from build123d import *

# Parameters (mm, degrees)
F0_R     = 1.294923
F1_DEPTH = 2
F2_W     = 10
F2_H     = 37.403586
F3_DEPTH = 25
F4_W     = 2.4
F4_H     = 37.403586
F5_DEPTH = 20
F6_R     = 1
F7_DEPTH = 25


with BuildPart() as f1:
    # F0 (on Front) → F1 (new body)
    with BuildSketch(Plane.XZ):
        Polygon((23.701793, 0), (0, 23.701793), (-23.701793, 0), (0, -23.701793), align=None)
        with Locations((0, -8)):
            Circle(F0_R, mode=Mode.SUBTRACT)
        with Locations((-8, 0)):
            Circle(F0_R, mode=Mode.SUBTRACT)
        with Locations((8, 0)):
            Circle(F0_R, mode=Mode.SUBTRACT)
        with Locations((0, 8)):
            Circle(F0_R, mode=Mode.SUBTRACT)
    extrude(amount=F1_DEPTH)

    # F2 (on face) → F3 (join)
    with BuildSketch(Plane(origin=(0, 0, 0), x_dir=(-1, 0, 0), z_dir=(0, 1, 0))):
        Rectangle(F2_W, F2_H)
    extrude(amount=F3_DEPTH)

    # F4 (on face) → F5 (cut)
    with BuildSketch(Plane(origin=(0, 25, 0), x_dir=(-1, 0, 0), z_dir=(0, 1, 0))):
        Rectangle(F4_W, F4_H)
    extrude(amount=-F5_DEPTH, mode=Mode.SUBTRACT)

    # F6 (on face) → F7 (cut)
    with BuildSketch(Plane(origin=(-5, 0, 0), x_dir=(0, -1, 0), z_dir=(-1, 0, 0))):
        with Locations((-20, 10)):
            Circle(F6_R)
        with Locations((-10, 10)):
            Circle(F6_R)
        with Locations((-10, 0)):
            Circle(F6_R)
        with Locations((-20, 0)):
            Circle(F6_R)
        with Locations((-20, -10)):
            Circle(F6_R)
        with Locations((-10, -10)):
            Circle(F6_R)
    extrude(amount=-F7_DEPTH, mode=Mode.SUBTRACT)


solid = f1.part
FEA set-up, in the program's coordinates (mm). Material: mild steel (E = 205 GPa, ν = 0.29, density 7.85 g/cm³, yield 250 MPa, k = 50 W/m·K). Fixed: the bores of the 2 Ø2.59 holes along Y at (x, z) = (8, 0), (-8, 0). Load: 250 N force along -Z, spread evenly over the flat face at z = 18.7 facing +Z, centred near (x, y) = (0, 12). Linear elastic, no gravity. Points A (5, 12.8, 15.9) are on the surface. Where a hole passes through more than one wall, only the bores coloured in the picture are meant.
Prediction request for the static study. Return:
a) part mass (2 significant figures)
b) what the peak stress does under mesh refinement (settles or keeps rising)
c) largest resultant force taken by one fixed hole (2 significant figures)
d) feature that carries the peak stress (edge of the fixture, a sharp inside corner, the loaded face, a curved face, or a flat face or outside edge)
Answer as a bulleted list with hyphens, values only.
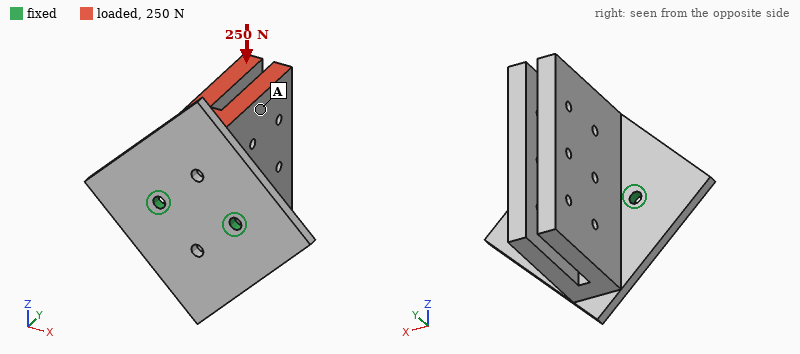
- 75 g
- keeps rising
- 130 N
- edge of the fixture
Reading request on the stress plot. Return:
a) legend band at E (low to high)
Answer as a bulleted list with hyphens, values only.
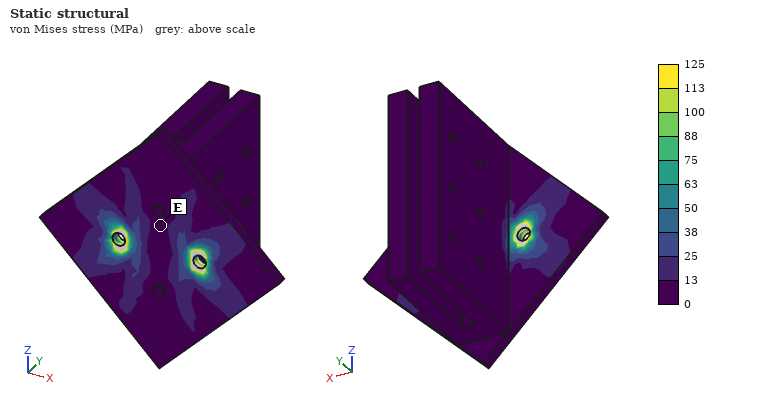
- 0 to 13 MPa
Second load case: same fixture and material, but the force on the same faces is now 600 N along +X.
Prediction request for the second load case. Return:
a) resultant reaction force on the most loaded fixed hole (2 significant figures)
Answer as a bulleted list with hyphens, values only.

- 930 N
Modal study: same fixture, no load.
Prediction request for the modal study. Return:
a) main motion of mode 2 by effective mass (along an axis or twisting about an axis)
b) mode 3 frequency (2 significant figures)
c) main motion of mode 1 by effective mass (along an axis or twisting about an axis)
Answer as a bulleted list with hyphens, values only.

- along X
- 6400 Hz
- along Z
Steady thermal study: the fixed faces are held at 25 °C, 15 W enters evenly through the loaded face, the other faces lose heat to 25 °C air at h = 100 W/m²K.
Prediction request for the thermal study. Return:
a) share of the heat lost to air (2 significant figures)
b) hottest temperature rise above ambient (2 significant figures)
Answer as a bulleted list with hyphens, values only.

- 57 %
- 35 K
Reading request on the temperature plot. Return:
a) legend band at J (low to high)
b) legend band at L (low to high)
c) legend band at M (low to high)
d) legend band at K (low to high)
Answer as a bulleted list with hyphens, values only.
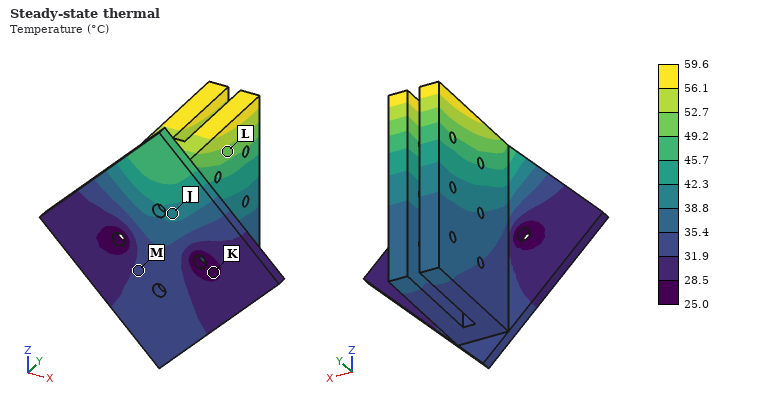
- 38.8 to 42.3 °C
- 49.2 to 52.7 °C
- 31.9 to 35.4 °C
- 25.0 to 28.5 °C
